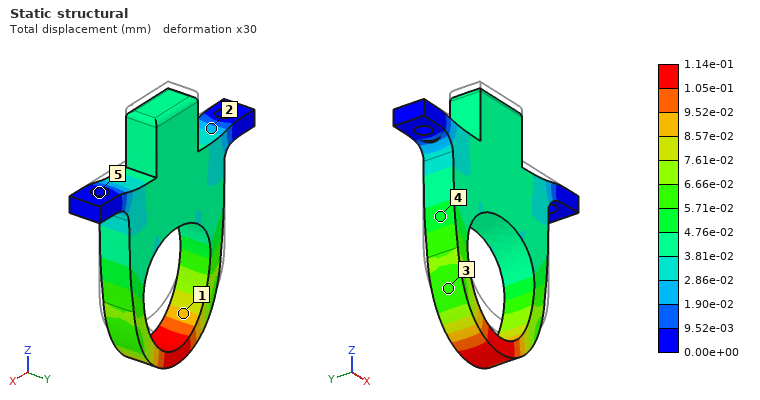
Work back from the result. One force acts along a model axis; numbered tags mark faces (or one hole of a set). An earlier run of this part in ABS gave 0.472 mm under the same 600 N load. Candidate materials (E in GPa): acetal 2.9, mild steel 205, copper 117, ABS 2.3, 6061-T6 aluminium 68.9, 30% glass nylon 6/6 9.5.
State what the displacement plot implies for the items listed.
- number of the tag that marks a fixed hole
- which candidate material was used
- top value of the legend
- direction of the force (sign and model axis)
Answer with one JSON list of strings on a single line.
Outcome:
["5", "30% glass nylon 6/6", "1.14e-01 mm", "-Z"]
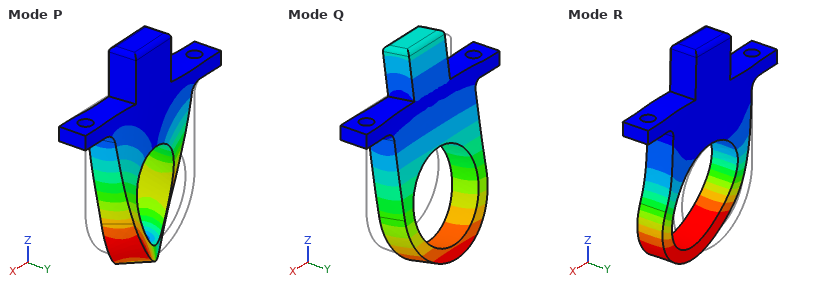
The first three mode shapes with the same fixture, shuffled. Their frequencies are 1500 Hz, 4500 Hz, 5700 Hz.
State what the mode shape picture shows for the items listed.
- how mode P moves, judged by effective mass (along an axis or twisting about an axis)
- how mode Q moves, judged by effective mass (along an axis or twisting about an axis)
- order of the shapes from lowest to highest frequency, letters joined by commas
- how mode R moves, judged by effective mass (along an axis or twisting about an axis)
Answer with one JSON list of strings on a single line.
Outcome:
["twisting about Z", "along Y", "Q, R, P", "along X"]
